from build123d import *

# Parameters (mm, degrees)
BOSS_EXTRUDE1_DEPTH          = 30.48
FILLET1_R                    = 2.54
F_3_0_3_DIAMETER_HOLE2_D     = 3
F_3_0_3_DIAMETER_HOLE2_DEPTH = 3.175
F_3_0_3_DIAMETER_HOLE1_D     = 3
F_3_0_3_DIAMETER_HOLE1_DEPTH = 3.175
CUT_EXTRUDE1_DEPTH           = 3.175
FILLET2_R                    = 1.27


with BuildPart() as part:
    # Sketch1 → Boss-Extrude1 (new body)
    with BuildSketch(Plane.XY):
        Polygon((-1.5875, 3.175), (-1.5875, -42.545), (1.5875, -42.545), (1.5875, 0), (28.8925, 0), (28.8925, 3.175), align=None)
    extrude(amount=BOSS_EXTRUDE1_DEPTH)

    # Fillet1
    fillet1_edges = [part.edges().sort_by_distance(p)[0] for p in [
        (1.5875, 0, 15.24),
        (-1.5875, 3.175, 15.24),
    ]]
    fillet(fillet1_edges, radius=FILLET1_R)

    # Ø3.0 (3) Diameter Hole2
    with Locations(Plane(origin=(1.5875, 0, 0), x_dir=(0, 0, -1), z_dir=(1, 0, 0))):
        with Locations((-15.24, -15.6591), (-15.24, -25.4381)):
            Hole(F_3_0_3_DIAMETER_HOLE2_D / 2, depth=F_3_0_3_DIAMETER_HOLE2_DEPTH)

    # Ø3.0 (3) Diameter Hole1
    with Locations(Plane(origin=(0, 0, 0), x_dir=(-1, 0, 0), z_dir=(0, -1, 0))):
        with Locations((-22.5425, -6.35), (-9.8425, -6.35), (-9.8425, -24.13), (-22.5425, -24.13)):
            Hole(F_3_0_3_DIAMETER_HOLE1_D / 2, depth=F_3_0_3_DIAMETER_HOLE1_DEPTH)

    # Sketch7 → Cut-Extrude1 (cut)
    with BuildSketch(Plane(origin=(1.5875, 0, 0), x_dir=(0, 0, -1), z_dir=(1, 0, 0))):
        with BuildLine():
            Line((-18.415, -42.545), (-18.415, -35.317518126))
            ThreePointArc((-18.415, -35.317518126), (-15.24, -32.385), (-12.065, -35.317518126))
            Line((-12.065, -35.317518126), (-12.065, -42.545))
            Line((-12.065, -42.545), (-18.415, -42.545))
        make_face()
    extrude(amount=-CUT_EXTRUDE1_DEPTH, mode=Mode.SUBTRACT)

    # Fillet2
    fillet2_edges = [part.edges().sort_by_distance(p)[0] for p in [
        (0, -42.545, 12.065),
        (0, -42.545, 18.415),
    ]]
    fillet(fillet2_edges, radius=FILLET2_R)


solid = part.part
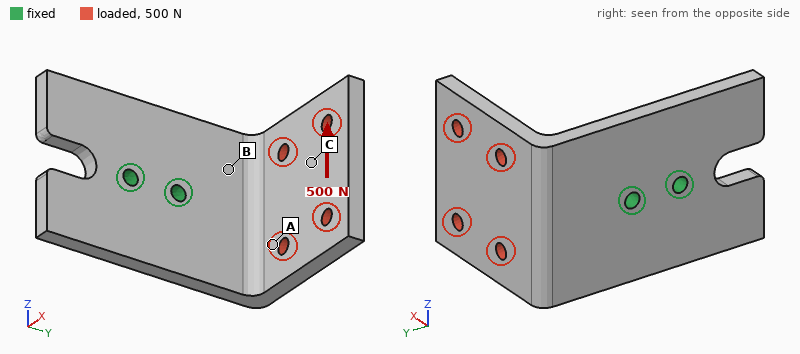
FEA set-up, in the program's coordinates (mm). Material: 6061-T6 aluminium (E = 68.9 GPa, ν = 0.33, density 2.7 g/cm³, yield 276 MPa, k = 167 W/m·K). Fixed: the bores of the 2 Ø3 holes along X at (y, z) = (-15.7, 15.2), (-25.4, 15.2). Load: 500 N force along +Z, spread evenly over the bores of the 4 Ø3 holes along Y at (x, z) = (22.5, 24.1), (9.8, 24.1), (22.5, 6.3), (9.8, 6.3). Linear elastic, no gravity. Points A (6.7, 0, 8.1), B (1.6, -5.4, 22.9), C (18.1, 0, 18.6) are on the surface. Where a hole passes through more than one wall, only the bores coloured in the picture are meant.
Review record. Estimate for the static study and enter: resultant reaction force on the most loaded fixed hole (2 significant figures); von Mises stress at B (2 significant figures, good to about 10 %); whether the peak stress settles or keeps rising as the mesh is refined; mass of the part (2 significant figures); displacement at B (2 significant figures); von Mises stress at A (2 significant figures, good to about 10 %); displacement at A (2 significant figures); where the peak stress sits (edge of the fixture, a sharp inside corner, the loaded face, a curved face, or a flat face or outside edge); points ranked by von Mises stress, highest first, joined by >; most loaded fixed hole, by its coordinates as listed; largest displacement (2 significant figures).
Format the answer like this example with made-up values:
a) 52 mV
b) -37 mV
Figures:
a) 1.2 kN
b) 92 MPa
c) keeps rising
d) 18 g
e) 0.090 mm
f) 54 MPa
g) 0.16 mm
h) edge of the fixture
i) B > A > C
j) (-15.7, 15.2)
k) 0.51 mm
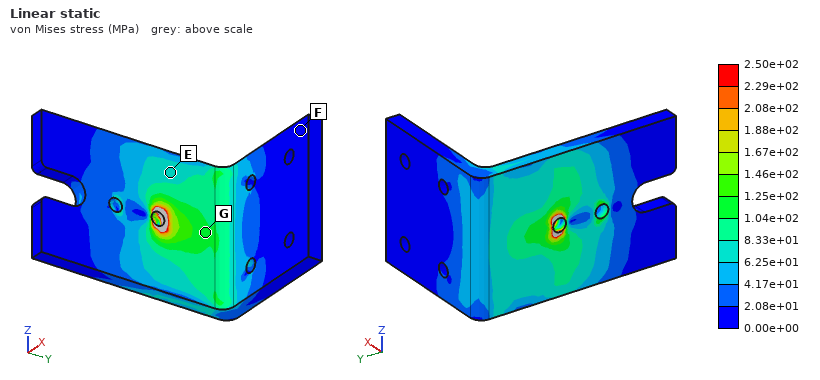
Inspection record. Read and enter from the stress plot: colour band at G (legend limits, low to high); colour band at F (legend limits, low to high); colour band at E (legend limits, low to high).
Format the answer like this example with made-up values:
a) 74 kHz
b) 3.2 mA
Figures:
a) 1.04e+02 to 1.25e+02 MPa
b) 0.00e+00 to 2.08e+01 MPa
c) 6.25e+01 to 8.33e+01 MPa
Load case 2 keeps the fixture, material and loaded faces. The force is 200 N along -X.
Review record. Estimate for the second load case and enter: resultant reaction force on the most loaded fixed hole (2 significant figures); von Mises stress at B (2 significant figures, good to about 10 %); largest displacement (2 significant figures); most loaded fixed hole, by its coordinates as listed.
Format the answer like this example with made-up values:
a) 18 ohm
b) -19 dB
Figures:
a) 350 N
b) 26 MPa
c) 0.19 mm
d) (-15.7, 15.2)
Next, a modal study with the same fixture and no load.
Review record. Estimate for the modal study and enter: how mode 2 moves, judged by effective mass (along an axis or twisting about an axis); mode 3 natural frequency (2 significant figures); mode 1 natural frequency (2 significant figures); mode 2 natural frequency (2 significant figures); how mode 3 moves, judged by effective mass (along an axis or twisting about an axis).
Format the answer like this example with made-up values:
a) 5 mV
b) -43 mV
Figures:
a) along Z
b) 4700 Hz
c) 1600 Hz
d) 2200 Hz
e) along X
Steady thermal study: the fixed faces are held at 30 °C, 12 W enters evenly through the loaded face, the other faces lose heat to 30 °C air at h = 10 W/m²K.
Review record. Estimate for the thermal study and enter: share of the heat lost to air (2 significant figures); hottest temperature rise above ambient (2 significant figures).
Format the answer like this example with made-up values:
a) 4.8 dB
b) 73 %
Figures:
a) 4.7 %
b) 27 K
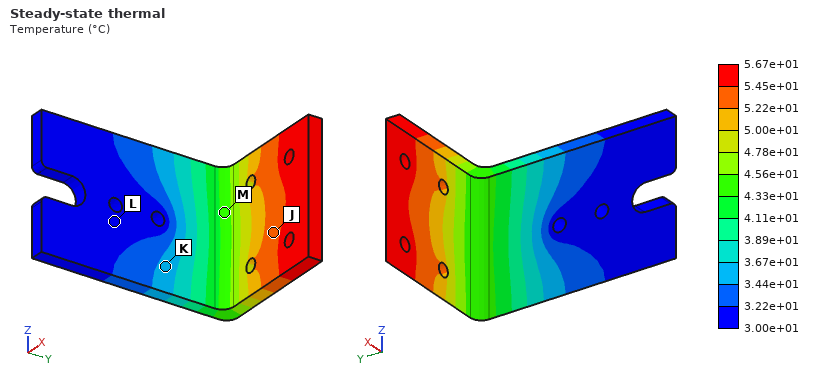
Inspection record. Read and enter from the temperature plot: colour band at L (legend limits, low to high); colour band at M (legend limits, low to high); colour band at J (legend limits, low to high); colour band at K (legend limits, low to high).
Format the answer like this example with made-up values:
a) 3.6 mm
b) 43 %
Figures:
a) 3.00e+01 to 3.22e+01 °C
b) 4.33e+01 to 4.56e+01 °C
c) 5.22e+01 to 5.45e+01 °C
d) 3.44e+01 to 3.67e+01 °C
